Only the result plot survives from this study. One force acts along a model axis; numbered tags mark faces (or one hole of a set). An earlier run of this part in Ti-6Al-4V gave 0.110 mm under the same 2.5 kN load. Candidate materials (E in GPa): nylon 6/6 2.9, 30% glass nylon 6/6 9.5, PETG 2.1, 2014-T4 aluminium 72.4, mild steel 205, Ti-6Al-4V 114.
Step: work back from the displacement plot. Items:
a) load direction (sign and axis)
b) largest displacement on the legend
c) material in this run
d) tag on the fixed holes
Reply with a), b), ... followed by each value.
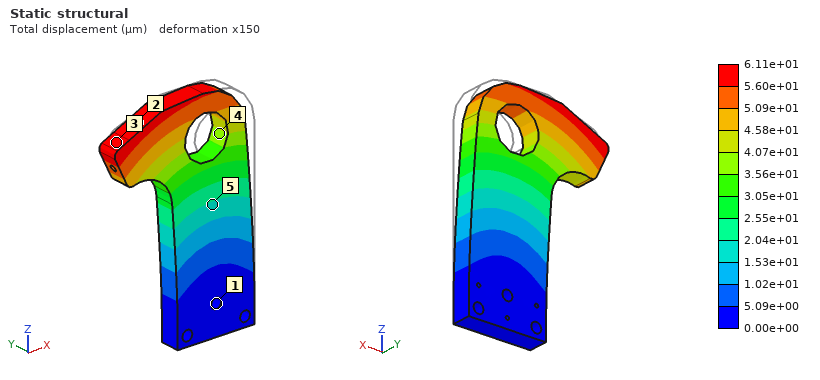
a) -X
b) 6.11e+01 µm
c) mild steel
d) 1
